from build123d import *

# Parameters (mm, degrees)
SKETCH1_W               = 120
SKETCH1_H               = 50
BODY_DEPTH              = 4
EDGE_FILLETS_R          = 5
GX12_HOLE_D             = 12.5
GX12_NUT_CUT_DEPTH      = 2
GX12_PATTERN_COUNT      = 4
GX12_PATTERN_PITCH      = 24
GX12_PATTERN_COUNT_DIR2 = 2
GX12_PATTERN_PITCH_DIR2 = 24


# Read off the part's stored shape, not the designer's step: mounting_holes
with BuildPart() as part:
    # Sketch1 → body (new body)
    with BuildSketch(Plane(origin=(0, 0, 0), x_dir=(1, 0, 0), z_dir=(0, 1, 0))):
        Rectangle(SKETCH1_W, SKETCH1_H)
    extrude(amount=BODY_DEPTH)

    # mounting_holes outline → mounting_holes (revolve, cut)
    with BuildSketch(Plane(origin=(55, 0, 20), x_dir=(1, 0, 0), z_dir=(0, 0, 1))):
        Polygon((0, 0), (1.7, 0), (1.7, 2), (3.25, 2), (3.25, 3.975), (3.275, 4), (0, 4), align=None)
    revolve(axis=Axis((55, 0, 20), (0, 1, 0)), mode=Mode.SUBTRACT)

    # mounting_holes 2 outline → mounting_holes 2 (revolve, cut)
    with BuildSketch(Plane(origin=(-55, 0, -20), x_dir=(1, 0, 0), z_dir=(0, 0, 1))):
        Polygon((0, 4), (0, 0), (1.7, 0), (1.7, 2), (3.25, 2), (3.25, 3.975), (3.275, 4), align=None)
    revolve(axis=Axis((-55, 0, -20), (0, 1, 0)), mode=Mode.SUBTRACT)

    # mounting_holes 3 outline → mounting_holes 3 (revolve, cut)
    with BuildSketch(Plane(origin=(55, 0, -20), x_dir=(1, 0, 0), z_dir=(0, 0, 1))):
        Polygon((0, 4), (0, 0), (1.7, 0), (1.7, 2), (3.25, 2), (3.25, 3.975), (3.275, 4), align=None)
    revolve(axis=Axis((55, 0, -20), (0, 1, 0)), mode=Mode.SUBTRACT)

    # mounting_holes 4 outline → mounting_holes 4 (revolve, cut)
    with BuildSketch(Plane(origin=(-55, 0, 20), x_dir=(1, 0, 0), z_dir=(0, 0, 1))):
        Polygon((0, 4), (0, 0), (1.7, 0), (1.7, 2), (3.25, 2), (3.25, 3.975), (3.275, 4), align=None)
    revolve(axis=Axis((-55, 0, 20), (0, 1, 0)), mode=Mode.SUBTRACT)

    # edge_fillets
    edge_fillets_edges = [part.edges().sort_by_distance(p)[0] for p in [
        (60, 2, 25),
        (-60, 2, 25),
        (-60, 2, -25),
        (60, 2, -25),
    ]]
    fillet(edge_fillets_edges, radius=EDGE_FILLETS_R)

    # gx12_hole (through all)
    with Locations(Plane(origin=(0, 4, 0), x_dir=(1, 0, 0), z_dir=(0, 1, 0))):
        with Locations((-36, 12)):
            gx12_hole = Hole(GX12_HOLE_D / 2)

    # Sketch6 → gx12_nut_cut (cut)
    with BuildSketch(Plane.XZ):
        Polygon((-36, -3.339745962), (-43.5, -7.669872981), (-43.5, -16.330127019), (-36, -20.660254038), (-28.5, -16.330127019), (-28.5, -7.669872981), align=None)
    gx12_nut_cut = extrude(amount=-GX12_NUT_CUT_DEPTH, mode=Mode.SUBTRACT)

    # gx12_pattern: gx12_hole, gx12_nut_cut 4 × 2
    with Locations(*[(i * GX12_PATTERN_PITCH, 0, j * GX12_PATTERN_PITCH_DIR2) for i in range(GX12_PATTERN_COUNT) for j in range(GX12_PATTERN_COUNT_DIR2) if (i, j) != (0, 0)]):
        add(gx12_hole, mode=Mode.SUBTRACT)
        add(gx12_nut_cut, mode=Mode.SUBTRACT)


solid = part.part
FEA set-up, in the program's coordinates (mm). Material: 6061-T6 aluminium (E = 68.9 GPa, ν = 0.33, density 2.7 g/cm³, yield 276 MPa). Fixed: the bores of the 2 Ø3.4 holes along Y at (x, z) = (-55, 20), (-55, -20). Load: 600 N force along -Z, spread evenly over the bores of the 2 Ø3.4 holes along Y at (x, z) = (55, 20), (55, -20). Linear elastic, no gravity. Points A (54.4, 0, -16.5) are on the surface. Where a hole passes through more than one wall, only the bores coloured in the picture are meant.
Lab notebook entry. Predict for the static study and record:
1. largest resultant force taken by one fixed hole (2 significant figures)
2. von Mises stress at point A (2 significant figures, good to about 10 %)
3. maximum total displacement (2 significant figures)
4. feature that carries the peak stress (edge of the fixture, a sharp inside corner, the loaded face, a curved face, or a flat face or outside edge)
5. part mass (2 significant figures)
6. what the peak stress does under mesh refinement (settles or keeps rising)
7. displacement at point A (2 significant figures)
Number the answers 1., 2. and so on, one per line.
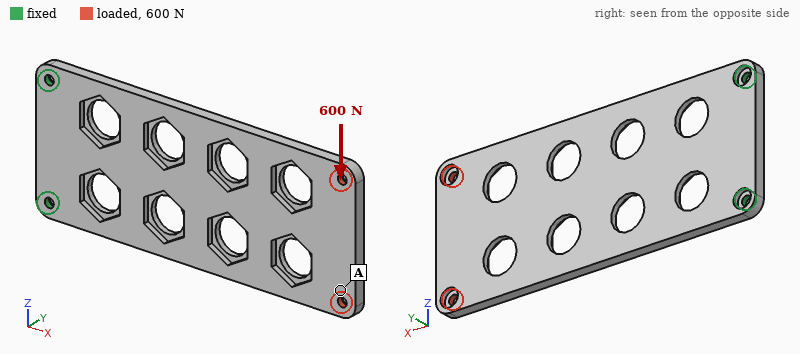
1. 1.6 kN
2. 17 MPa
3. 0.28 mm
4. edge of the fixture
5. 50 g
6. keeps rising
7. 0.24 mm
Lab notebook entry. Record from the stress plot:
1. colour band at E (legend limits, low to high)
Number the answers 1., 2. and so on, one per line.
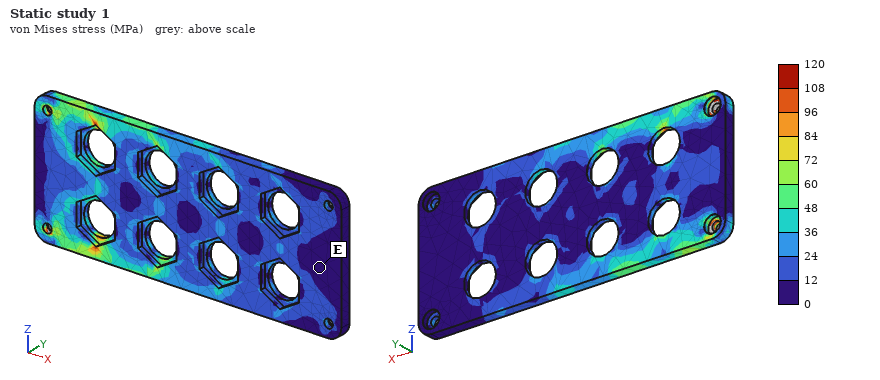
1. 0 to 12 MPa
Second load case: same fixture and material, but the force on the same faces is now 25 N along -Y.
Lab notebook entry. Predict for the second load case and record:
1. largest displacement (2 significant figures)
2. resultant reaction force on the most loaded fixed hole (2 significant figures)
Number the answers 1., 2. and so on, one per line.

1. 1.3 mm
2. 13 N
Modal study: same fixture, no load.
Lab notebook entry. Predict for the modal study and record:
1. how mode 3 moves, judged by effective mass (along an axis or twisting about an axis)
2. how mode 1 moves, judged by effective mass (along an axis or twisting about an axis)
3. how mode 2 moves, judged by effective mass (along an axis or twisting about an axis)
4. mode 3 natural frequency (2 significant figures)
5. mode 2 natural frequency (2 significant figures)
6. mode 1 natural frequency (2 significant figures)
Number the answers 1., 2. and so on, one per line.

1. along Y
2. along Y
3. twisting about X
4. 1200 Hz
5. 1000 Hz
6. 190 Hz
